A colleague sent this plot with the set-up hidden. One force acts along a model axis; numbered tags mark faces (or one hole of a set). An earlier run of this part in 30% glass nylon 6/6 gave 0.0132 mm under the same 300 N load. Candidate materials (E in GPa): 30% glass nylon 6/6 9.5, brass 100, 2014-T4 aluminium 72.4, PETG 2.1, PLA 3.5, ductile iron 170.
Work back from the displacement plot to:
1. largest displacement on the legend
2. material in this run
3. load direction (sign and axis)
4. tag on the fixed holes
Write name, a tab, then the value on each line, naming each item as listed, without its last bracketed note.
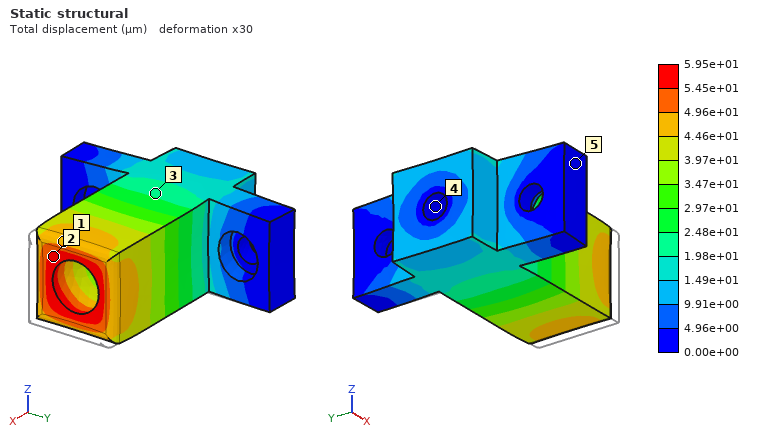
largest displacement on the legend	5.95e+01 µm
material in this run	PETG
load direction	-X
tag on the fixed holes	4
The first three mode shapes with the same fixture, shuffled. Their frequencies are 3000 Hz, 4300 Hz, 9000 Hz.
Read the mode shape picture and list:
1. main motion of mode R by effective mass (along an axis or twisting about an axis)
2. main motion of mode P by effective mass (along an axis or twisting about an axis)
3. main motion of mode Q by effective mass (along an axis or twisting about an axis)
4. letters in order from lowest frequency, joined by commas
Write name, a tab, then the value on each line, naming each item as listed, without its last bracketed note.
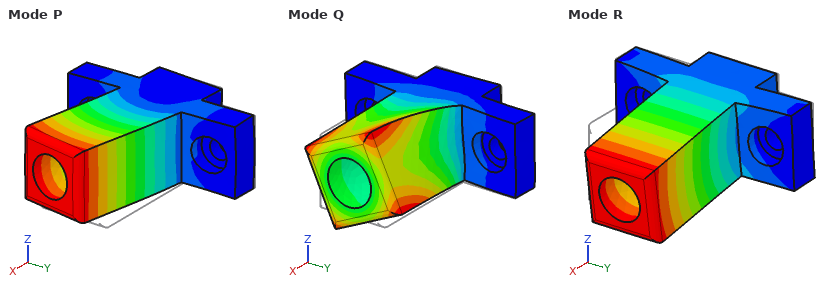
main motion of mode R by effective mass	along Z
main motion of mode P by effective mass	along Y
main motion of mode Q by effective mass	twisting about X
letters in order from lowest frequency, joined by commas	R, P, Q
